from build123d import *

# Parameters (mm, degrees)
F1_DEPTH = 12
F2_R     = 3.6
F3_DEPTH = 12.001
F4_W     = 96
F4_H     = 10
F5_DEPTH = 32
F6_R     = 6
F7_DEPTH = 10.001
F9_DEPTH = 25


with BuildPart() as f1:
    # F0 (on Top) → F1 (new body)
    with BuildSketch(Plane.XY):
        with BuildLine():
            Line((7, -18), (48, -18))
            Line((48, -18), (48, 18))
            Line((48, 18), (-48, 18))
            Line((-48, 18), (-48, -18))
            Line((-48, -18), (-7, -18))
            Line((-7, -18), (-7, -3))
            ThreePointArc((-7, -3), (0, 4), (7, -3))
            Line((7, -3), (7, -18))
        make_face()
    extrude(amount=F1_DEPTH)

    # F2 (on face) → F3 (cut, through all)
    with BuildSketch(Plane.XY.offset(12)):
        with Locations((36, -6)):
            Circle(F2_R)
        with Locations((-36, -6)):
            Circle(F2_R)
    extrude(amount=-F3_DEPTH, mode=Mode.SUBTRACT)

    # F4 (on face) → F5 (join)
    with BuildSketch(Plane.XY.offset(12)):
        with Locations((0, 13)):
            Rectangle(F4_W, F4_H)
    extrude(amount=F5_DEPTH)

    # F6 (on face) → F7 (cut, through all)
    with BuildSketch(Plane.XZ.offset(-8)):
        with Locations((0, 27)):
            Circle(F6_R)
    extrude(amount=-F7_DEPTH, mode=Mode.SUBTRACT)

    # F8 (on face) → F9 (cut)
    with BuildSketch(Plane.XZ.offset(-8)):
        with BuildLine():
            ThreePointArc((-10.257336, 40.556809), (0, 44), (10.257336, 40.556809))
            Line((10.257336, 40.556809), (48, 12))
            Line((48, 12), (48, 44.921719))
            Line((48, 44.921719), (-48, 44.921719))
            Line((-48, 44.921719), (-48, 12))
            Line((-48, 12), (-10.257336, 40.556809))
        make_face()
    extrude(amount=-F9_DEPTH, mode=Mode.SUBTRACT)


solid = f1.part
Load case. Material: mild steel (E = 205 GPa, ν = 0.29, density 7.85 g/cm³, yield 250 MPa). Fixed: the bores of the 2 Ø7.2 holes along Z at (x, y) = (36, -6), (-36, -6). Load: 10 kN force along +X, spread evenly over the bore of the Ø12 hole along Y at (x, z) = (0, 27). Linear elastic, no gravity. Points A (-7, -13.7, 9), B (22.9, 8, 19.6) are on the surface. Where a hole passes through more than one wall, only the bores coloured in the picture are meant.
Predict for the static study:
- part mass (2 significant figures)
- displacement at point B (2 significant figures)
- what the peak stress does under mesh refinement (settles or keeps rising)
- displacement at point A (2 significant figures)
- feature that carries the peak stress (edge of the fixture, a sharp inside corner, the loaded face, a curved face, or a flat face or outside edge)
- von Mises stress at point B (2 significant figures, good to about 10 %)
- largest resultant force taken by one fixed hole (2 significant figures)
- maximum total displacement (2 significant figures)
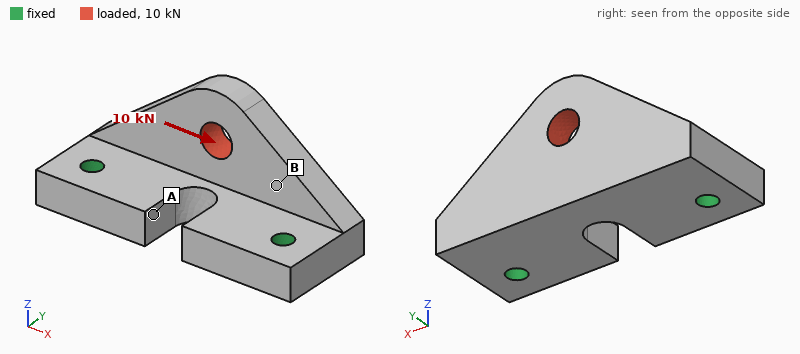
420 g
9.5 µm
keeps rising
2.7 µm
edge of the fixture
36 MPa
6.1 kN
17 µm
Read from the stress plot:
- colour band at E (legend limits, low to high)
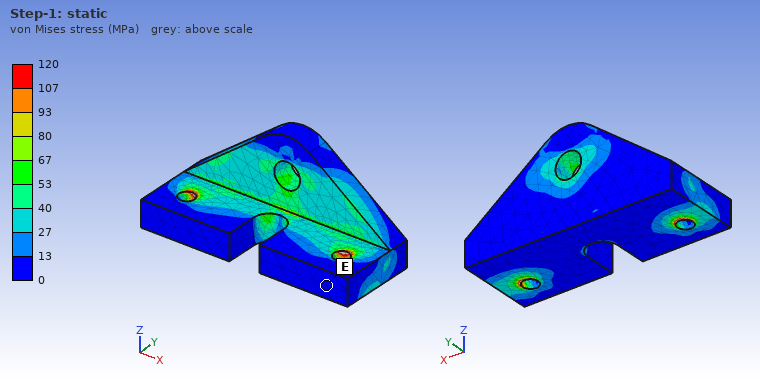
0 to 13 MPa
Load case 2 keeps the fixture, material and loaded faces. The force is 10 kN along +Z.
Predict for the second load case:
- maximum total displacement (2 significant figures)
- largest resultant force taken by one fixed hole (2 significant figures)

57 µm
5.0 kN
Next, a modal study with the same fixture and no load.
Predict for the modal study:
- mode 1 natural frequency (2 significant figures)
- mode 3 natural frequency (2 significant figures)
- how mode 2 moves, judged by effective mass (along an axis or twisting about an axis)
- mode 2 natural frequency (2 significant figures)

4900 Hz
10000 Hz
along Z
9400 Hz
